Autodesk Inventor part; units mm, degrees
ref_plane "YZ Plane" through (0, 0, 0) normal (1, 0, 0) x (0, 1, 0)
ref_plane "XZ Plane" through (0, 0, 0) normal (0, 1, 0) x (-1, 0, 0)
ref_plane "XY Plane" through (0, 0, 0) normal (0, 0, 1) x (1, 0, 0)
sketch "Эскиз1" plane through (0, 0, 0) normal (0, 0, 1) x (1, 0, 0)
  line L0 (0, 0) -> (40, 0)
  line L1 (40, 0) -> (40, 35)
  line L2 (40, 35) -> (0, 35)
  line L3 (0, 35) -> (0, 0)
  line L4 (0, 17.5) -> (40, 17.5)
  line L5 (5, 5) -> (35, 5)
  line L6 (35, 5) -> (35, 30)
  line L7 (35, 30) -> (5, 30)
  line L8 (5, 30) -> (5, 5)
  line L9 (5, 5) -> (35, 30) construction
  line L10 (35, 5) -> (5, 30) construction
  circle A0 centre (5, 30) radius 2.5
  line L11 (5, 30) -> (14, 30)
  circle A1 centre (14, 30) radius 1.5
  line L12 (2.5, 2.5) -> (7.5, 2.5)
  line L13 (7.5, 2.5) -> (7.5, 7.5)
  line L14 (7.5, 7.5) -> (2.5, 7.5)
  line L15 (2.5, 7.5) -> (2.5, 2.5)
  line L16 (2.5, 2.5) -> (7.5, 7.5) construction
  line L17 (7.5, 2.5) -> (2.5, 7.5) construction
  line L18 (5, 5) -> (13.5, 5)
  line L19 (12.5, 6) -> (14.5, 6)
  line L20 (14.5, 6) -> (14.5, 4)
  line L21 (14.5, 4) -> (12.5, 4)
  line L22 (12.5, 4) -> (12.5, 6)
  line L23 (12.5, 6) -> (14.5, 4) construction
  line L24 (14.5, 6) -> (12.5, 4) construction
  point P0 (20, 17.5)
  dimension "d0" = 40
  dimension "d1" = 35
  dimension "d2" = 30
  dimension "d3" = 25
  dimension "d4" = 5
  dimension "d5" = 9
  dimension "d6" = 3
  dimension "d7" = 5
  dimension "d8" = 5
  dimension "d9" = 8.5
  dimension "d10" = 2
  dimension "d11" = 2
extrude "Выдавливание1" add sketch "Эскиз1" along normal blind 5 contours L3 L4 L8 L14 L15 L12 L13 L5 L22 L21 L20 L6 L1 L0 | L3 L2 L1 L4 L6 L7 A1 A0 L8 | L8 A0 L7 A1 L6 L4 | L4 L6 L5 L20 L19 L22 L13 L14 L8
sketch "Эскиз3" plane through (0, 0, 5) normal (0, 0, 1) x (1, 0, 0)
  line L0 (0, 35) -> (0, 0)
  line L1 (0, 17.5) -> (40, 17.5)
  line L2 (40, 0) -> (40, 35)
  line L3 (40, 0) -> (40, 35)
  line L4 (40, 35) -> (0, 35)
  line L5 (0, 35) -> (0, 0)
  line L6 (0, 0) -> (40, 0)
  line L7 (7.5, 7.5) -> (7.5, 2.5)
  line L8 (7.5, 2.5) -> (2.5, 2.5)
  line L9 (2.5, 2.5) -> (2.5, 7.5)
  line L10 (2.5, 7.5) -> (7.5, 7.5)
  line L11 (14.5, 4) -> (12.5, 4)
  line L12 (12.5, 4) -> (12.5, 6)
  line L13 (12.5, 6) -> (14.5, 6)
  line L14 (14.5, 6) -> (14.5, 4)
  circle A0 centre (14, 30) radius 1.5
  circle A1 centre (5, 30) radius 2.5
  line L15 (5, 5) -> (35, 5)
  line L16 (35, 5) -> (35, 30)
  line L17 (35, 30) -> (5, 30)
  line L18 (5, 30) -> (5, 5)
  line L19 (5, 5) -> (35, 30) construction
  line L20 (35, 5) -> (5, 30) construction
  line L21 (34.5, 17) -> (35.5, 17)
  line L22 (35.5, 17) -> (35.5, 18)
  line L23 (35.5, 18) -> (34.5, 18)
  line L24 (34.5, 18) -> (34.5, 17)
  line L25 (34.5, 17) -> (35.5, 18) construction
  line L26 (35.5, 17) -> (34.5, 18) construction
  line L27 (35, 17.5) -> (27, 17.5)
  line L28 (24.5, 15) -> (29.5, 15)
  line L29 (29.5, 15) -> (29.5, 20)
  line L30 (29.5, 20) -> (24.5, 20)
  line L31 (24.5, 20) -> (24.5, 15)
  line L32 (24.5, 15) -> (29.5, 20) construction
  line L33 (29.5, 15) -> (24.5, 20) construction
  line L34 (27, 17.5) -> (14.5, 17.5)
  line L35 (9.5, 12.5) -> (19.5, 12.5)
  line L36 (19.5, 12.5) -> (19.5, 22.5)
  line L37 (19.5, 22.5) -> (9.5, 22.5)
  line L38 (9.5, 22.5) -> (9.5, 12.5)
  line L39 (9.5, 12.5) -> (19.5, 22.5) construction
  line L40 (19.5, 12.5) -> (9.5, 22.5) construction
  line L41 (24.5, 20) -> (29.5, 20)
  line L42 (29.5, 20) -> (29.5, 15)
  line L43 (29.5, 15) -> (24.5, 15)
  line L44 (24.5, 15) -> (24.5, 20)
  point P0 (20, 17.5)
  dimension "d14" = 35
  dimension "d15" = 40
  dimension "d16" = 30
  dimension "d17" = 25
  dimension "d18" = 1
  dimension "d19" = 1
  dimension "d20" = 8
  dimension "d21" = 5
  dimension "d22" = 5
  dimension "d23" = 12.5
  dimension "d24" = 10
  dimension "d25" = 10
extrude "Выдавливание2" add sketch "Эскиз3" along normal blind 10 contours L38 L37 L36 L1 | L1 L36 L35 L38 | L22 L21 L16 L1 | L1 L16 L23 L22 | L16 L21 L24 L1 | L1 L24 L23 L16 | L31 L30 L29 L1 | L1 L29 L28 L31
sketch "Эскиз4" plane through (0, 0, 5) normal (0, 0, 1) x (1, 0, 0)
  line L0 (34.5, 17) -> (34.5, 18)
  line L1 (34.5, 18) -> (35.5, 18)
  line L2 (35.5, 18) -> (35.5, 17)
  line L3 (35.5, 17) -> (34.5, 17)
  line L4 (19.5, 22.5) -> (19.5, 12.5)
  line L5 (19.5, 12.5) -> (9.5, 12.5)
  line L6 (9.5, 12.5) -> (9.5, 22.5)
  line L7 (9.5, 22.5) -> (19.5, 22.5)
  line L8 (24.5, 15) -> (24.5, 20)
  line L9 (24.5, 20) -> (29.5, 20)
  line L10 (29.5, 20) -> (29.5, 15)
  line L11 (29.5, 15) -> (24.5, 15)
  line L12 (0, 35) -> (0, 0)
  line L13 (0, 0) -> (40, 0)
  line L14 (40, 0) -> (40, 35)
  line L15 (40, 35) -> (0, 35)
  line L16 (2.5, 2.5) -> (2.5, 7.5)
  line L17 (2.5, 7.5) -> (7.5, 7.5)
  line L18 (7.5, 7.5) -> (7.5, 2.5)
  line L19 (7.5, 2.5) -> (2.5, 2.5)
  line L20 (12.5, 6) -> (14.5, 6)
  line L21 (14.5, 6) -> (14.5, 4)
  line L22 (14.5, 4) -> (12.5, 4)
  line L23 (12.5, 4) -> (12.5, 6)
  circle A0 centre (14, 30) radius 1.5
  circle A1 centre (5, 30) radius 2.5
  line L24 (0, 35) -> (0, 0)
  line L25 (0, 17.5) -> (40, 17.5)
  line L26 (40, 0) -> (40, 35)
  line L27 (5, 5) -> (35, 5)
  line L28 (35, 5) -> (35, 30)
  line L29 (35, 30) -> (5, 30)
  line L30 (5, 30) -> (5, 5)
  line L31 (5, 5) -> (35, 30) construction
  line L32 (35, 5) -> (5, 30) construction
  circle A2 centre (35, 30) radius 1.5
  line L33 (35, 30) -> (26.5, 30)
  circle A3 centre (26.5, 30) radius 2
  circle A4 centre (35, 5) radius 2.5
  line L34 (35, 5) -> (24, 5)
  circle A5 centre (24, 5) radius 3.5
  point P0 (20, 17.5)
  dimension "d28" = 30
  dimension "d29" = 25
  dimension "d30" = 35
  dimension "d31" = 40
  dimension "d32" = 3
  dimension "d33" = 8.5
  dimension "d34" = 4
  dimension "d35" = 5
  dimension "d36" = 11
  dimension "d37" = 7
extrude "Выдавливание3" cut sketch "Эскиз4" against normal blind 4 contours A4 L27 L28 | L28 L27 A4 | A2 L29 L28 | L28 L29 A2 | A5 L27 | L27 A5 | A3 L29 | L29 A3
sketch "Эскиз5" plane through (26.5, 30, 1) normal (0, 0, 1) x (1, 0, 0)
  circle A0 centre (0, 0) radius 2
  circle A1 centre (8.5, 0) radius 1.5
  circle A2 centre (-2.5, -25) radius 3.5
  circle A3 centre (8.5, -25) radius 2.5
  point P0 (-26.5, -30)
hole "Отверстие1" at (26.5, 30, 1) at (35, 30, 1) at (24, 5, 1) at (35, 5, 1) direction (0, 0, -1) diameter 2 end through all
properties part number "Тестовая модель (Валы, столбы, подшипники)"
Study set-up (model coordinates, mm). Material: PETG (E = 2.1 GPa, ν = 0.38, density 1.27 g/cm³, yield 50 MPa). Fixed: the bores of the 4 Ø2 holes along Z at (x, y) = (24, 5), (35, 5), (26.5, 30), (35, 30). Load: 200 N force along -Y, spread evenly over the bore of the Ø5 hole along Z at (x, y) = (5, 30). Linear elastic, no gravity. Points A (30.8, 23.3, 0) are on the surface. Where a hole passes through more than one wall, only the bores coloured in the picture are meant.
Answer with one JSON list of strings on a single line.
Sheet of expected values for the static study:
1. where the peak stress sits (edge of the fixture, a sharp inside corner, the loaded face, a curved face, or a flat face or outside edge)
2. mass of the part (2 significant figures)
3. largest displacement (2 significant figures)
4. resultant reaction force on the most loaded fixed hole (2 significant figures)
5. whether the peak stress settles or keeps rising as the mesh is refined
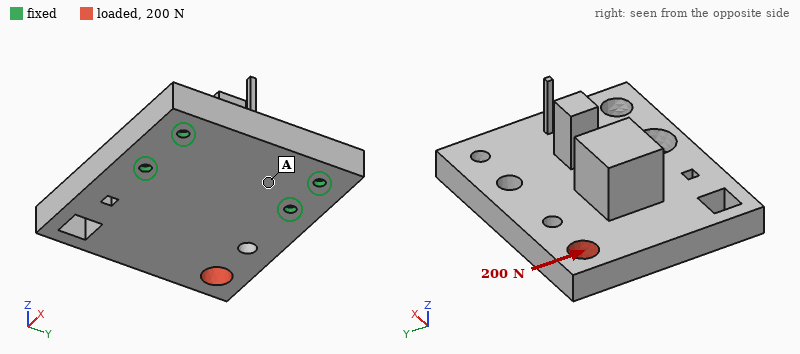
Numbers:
["edge of the fixture", "9.7 g", "0.15 mm", "140 N", "keeps rising"]
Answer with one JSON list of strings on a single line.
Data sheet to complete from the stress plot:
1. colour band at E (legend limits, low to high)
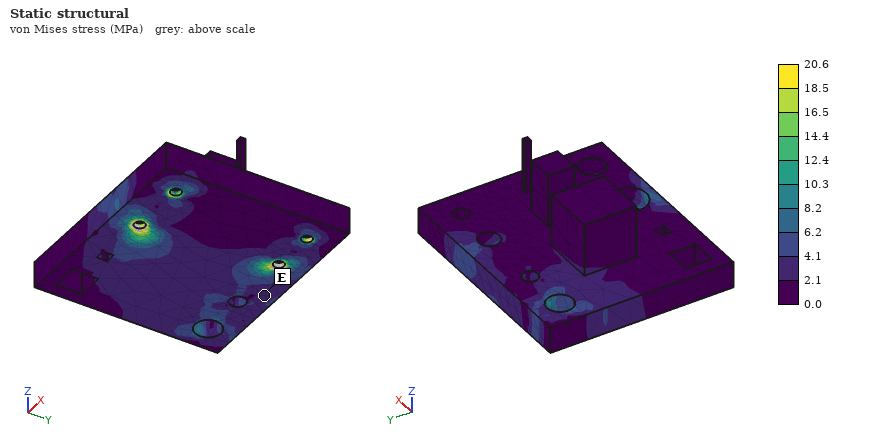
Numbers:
["2.1 to 4.1 MPa"]
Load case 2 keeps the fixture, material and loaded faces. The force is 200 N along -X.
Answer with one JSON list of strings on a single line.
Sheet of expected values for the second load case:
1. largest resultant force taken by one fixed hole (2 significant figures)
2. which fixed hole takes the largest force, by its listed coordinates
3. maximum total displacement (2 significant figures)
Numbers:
["120 N", "(26.5, 30)", "0.14 mm"]
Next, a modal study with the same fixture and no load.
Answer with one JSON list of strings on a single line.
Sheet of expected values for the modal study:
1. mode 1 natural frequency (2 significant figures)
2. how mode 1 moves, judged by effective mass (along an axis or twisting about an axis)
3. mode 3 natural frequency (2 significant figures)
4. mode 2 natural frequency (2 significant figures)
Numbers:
["910 Hz", "along Z", "2000 Hz", "2000 Hz"]
